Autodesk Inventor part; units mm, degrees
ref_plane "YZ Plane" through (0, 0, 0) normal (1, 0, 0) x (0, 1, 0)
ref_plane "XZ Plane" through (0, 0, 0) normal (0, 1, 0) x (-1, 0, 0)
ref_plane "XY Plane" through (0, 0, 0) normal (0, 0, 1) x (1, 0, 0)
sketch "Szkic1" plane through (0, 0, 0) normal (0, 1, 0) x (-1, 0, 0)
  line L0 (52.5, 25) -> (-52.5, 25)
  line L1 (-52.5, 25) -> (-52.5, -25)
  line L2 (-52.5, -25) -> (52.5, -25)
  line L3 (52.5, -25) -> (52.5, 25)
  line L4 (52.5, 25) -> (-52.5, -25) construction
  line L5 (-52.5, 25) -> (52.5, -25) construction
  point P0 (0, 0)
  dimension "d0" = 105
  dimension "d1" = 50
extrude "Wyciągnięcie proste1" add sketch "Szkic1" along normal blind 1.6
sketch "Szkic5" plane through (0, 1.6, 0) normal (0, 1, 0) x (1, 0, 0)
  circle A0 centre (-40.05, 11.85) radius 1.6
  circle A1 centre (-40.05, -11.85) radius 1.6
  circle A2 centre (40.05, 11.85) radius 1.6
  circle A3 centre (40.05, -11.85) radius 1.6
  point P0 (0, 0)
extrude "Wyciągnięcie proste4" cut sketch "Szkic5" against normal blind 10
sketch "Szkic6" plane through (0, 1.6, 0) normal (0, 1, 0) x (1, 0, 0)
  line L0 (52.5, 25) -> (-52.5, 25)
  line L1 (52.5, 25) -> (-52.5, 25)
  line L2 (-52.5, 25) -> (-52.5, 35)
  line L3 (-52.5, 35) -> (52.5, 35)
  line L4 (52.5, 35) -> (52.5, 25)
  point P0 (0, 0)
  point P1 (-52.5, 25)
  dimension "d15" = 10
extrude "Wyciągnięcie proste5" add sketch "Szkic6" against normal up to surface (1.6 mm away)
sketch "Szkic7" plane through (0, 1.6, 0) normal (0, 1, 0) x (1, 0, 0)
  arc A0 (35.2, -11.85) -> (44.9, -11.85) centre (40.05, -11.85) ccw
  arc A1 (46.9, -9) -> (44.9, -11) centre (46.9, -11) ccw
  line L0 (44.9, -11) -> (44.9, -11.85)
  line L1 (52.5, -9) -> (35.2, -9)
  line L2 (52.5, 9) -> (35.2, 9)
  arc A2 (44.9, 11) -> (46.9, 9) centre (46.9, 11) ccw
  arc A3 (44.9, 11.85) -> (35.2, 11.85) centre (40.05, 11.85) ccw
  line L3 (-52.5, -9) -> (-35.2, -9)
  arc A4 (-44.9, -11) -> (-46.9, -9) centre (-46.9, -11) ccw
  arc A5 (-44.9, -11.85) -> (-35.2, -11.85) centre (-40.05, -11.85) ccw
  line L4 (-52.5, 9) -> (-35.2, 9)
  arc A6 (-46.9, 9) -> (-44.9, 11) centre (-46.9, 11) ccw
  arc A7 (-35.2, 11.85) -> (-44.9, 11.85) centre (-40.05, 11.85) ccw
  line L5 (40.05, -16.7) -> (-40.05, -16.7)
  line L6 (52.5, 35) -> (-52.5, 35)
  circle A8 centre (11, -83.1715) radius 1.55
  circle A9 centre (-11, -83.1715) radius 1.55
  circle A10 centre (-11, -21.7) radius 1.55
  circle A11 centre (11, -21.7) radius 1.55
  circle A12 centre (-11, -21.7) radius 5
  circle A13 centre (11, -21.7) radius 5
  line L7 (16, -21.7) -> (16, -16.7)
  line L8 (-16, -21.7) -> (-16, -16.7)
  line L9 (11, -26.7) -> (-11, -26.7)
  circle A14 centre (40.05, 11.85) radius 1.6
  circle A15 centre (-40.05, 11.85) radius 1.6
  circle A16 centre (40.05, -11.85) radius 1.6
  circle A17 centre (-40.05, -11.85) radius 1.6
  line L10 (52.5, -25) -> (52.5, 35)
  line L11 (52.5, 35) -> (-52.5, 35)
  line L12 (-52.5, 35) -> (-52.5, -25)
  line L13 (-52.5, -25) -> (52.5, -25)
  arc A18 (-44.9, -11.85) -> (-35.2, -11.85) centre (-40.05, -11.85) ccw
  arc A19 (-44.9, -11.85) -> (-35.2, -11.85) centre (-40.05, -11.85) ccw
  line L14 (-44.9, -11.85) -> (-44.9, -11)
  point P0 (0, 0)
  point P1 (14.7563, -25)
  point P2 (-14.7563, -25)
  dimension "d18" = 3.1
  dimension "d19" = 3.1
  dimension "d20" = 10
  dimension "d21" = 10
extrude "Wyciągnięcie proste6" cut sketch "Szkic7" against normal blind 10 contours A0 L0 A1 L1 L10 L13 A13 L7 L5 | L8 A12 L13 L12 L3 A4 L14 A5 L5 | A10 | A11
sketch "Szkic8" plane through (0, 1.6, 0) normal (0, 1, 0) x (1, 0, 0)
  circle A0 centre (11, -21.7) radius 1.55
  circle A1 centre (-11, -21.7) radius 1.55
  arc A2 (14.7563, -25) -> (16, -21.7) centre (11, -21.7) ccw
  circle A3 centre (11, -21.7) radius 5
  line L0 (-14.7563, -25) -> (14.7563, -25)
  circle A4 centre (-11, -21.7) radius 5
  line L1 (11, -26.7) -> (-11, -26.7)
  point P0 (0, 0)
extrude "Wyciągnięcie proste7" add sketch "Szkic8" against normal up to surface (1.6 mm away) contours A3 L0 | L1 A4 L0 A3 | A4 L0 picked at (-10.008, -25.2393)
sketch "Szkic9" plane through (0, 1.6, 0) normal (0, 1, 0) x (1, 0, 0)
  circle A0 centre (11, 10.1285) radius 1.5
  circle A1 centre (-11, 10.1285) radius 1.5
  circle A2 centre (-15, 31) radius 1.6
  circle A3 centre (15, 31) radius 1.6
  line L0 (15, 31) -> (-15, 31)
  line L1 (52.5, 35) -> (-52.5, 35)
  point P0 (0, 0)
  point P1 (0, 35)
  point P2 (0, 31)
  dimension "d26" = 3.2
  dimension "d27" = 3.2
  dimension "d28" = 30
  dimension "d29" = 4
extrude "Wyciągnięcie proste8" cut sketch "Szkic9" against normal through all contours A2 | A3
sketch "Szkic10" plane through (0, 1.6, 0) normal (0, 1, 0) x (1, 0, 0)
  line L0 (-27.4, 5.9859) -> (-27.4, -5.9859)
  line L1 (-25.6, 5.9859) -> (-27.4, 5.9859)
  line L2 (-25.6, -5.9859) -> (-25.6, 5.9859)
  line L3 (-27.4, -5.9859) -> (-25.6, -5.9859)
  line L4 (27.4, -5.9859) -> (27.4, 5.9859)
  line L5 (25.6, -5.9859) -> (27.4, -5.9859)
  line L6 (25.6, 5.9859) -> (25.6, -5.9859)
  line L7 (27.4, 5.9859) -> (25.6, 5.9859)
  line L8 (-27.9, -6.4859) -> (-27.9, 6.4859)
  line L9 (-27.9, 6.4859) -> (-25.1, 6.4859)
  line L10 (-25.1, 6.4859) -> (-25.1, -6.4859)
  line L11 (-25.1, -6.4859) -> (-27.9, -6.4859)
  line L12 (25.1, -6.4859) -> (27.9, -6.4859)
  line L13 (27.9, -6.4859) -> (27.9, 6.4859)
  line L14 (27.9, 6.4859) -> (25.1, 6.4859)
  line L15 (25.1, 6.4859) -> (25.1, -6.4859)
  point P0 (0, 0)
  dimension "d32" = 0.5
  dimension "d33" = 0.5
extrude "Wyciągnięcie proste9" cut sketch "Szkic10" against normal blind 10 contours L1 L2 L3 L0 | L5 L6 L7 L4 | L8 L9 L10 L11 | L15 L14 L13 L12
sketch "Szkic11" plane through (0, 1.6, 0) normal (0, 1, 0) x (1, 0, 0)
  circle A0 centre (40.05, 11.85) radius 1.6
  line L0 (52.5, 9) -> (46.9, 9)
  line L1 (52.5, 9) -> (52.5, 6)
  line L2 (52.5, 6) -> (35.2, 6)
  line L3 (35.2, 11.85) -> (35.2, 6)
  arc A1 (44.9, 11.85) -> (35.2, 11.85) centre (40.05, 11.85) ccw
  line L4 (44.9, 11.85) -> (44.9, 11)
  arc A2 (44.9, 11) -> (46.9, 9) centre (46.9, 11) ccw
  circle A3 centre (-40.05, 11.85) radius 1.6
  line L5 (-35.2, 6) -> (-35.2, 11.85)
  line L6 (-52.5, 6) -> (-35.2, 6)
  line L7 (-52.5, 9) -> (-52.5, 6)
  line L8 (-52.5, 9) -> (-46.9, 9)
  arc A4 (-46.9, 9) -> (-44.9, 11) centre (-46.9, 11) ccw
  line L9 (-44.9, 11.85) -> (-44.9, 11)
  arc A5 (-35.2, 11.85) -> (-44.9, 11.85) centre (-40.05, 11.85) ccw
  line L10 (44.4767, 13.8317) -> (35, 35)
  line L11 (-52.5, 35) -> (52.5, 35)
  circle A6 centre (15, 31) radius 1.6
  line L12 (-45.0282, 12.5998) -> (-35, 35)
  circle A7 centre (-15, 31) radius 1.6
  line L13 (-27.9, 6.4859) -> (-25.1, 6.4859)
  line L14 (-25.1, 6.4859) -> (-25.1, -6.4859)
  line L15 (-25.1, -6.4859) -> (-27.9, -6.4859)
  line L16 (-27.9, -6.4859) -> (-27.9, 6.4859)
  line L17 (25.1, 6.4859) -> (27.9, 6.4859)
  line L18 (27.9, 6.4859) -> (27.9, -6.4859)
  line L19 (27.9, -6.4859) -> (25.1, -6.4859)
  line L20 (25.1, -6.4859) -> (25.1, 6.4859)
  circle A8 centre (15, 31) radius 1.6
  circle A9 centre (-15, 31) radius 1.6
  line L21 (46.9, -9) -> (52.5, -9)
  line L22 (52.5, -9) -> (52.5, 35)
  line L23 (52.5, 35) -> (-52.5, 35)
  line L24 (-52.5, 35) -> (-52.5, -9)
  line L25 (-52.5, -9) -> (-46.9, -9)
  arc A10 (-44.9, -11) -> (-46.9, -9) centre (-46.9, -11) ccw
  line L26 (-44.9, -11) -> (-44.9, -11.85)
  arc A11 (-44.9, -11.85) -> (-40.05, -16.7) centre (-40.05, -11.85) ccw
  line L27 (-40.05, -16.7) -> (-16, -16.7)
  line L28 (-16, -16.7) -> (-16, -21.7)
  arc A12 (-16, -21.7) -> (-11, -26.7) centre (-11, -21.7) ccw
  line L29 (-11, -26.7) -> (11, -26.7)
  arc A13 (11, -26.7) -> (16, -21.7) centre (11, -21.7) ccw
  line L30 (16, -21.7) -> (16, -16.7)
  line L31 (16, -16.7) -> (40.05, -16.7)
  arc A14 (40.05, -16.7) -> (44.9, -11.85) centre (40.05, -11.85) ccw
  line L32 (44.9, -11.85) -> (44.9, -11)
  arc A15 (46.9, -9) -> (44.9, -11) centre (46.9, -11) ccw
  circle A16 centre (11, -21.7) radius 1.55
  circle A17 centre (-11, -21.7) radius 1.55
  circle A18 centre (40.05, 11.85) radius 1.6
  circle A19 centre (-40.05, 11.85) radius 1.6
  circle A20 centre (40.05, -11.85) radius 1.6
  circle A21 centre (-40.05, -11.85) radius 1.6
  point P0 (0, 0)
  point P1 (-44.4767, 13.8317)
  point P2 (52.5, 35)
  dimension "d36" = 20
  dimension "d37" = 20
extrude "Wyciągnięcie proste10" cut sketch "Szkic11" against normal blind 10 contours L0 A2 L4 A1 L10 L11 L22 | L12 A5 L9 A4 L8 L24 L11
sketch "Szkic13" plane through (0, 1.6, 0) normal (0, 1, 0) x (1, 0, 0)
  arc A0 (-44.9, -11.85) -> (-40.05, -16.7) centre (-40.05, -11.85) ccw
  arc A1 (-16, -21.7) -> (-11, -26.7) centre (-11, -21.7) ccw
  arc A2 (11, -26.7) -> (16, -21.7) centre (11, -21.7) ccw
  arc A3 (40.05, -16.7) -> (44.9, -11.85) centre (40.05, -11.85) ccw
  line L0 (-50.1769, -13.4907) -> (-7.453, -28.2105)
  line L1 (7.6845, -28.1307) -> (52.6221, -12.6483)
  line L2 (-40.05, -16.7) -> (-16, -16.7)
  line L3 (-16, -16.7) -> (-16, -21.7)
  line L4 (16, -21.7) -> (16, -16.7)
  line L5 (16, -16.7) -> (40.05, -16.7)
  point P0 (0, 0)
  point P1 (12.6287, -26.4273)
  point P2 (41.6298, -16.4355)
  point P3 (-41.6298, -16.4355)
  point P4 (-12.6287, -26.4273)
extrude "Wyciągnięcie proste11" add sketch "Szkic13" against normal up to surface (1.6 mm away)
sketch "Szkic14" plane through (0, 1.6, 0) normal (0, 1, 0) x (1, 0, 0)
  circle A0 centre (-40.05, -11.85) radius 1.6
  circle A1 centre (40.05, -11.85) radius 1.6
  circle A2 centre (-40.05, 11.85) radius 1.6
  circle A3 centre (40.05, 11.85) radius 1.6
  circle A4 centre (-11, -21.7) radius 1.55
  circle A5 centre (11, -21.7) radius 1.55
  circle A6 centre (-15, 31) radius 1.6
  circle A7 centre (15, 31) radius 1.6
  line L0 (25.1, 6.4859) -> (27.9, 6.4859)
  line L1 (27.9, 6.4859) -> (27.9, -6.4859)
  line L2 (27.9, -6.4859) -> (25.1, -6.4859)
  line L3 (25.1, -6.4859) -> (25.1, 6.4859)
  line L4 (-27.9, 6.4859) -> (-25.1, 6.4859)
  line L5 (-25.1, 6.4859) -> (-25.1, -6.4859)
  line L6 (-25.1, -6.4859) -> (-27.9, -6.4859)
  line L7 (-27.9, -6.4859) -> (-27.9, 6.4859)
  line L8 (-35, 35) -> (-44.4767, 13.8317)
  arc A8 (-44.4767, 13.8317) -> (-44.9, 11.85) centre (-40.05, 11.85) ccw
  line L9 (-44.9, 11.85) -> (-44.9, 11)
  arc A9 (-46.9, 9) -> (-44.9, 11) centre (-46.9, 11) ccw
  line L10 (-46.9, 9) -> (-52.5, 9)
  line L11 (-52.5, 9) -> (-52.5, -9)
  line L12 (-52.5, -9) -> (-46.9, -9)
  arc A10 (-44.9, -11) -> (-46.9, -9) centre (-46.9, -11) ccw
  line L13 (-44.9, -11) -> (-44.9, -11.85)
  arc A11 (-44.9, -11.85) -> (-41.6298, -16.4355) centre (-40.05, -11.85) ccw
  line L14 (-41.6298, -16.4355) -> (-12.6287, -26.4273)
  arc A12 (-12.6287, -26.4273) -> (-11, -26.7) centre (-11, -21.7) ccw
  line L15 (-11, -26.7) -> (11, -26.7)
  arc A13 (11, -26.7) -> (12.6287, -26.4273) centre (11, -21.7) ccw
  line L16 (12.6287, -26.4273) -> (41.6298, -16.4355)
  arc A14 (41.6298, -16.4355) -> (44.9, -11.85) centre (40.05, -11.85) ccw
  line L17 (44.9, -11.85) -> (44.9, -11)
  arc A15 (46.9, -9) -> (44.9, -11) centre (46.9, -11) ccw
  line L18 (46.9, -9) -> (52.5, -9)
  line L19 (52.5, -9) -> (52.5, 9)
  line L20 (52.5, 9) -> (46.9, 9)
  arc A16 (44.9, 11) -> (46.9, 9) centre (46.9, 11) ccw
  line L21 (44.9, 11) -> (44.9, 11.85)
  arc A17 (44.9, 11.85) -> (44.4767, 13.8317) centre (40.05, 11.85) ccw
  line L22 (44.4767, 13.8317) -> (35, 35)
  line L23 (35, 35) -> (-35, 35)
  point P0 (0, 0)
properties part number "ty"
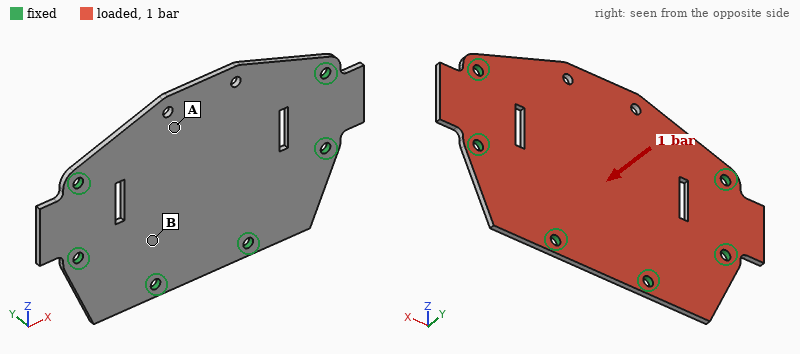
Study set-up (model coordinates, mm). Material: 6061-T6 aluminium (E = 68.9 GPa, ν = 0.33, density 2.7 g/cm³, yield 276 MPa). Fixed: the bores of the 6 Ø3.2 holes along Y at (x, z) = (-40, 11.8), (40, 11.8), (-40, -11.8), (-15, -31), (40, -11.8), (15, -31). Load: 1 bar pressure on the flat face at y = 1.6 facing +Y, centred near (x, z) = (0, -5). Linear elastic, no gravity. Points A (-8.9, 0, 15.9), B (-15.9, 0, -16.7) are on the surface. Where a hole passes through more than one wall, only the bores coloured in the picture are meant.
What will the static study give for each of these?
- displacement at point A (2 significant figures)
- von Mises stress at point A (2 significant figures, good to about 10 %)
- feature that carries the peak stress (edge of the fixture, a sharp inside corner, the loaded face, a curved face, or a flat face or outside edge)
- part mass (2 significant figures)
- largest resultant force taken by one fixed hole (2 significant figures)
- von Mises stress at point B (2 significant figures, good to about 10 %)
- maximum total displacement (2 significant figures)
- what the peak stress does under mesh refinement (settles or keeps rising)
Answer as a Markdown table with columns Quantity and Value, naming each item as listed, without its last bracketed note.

| Quantity | Value |
|---|---|
| displacement at point A | 0.43 mm |
| von Mises stress at point A | 50 MPa |
| feature that carries the peak stress | edge of the fixture |
| part mass | 22 g |
| largest resultant force taken by one fixed hole | 110 N |
| von Mises stress at point B | 25 MPa |
| maximum total displacement | 0.60 mm |
| what the peak stress does under mesh refinement | keeps rising |
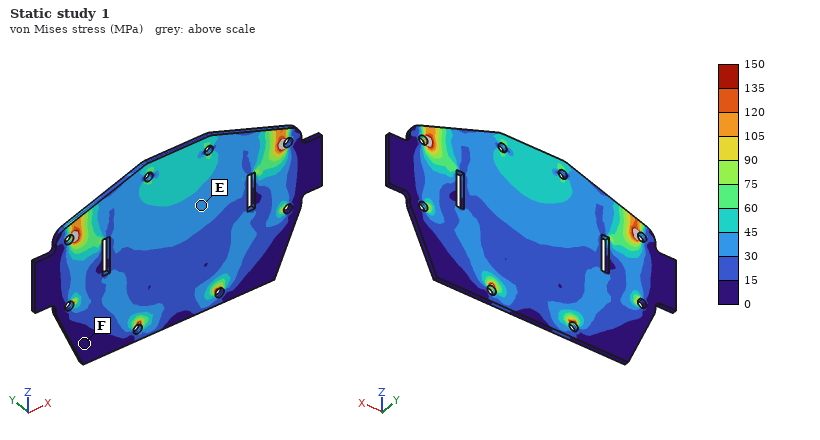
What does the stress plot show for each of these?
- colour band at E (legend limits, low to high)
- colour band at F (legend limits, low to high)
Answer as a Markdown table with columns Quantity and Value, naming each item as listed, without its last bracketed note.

| Quantity | Value |
|---|---|
| colour band at E | 30 to 45 MPa |
| colour band at F | 0 to 15 MPa |
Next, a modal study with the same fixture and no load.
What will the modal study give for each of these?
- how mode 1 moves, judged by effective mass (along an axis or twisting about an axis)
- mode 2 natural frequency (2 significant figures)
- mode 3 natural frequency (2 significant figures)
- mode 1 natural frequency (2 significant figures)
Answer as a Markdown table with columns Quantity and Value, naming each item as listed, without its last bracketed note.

| Quantity | Value |
|---|---|
| how mode 1 moves, judged by effective mass | along Y |
| mode 2 natural frequency | 3200 Hz |
| mode 3 natural frequency | 3600 Hz |
| mode 1 natural frequency | 1300 Hz |
